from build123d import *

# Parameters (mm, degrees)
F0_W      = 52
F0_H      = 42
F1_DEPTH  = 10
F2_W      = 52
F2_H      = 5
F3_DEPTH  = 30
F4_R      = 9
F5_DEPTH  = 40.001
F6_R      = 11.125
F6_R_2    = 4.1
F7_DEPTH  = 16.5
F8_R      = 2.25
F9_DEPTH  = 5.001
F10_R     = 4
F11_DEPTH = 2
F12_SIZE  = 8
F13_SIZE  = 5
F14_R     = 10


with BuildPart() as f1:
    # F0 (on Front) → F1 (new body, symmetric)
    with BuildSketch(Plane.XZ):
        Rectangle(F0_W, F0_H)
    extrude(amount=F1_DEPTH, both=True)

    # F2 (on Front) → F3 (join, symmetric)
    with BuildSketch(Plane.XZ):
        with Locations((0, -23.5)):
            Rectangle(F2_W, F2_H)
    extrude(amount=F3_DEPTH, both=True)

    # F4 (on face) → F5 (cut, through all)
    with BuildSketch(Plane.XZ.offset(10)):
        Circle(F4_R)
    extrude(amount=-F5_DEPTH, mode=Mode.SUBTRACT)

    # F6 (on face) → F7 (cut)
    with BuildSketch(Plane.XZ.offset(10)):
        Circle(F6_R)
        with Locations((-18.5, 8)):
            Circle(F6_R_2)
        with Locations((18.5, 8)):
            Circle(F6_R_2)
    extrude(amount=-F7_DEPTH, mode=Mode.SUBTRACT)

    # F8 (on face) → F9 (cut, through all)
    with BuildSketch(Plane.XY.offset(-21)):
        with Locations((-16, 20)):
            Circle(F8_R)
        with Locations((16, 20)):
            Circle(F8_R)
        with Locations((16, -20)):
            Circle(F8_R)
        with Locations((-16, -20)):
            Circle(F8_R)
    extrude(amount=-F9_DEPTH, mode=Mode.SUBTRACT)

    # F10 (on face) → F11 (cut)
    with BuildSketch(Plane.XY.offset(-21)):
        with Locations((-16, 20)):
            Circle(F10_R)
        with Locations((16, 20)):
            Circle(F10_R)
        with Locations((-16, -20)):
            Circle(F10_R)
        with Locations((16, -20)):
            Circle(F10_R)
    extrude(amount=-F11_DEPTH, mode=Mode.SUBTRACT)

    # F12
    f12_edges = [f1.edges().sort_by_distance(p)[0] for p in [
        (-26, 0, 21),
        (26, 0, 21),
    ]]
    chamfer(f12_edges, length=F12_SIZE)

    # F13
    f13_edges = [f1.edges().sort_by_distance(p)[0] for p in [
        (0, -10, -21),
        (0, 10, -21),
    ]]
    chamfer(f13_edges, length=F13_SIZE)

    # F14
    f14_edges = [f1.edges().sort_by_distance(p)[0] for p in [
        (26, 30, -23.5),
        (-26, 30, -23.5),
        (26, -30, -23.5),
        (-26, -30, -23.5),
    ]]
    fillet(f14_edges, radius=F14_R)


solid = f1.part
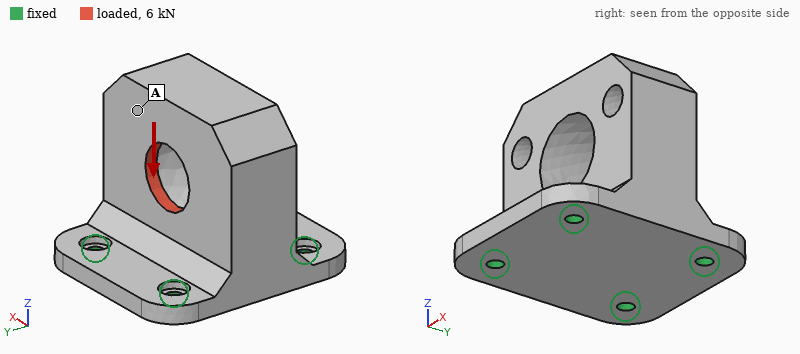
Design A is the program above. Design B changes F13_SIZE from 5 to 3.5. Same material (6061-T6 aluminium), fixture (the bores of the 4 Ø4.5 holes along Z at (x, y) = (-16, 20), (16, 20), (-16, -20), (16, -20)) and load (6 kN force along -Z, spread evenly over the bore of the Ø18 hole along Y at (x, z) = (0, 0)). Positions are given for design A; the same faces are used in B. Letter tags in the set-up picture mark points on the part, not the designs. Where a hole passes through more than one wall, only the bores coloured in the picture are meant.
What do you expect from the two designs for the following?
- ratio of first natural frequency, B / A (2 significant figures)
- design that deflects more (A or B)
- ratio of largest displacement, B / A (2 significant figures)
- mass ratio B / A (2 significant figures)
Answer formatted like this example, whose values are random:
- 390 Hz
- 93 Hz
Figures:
- 0.93
- B
- 1.2
- 0.99
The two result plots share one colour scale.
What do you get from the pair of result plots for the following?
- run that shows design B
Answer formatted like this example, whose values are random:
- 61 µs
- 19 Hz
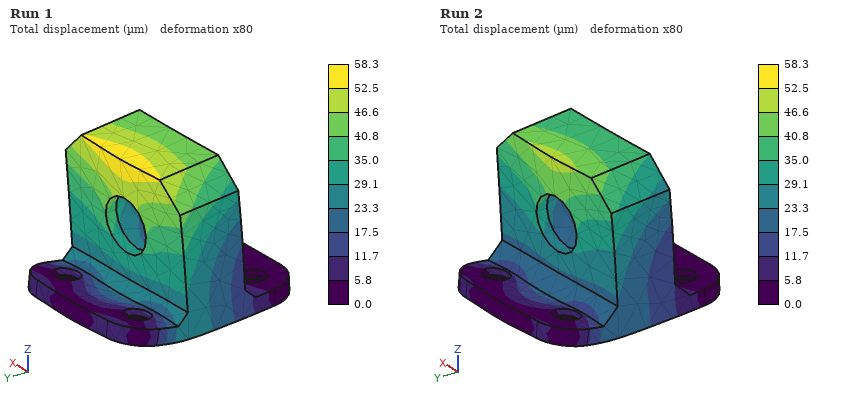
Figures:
- Run 1
